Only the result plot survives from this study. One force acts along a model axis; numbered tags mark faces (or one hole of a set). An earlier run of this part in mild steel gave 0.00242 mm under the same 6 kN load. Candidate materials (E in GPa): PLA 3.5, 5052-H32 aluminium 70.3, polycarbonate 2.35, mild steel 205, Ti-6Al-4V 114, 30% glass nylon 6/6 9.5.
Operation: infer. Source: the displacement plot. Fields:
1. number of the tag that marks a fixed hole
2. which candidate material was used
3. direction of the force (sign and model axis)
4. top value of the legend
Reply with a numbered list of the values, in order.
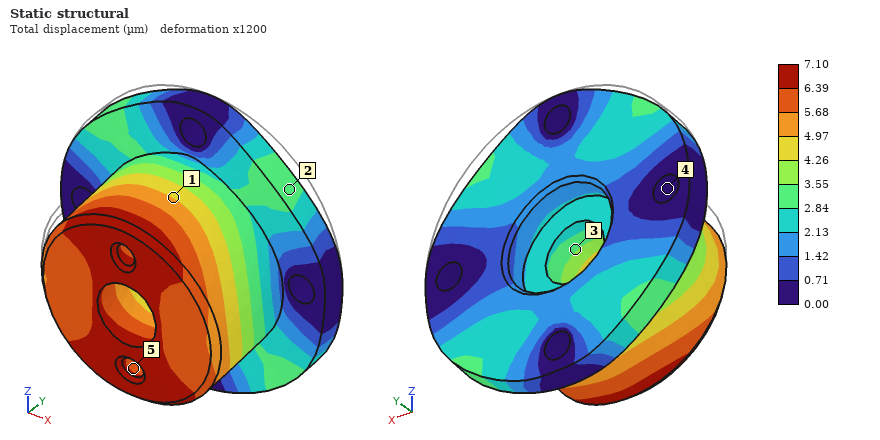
1. 4
2. 5052-H32 aluminium
3. -Z
4. 7.10 µm
